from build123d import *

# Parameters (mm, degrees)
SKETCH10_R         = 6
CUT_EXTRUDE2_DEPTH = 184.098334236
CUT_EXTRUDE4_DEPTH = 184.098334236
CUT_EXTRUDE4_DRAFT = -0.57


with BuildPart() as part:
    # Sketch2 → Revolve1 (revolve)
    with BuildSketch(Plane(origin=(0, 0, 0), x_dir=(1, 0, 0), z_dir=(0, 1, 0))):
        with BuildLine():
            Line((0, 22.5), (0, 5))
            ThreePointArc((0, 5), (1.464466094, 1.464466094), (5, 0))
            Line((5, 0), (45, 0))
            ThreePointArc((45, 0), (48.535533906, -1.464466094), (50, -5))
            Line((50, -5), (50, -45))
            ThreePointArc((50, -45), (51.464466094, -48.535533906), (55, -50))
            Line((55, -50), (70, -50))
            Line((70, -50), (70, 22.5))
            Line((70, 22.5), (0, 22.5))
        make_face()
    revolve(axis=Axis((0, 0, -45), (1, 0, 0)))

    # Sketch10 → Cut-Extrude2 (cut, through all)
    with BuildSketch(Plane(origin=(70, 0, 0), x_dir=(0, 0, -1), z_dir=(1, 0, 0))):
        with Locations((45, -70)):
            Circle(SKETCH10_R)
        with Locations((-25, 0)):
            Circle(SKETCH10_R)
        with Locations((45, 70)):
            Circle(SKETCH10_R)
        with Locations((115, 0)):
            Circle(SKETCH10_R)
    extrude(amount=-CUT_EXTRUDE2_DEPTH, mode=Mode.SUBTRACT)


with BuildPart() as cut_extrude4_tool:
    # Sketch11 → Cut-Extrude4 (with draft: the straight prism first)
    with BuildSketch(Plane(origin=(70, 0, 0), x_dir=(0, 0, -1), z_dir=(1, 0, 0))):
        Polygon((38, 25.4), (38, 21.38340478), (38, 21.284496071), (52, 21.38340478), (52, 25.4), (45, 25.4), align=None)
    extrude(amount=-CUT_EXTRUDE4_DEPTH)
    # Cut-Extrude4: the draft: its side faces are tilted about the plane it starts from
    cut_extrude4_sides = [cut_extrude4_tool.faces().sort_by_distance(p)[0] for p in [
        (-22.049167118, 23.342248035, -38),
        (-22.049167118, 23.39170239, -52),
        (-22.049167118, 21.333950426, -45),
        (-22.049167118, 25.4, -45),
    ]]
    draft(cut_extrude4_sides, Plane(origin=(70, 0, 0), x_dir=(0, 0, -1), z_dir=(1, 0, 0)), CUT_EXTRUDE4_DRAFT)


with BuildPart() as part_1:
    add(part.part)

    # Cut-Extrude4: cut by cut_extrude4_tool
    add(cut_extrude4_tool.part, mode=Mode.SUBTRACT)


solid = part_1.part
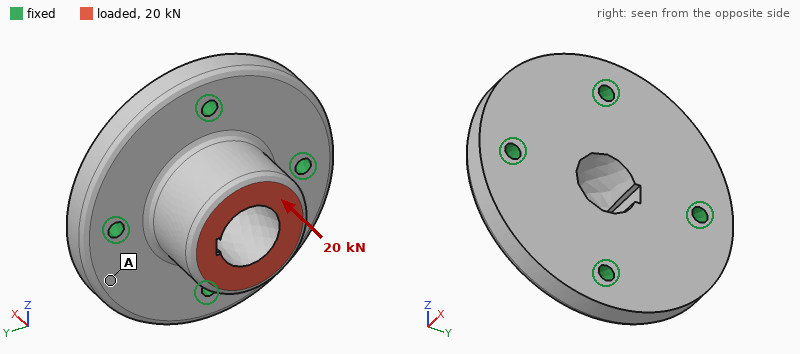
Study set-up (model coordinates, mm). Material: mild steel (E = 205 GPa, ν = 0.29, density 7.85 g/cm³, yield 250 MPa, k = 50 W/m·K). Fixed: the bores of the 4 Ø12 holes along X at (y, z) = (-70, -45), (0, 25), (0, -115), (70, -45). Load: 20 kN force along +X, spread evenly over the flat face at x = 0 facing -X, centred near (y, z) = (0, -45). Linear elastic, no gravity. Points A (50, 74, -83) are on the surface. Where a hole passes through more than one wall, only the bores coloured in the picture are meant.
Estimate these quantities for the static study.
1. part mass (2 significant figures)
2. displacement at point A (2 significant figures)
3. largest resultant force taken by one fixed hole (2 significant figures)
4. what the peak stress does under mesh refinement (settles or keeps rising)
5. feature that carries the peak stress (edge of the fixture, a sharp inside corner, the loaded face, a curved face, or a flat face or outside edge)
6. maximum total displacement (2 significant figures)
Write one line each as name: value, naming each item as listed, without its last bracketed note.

part mass: 6.0 kg
displacement at point A: 0.85 µm
largest resultant force taken by one fixed hole: 5.3 kN
what the peak stress does under mesh refinement: keeps rising
feature that carries the peak stress: edge of the fixture
maximum total displacement: 5.5 µm
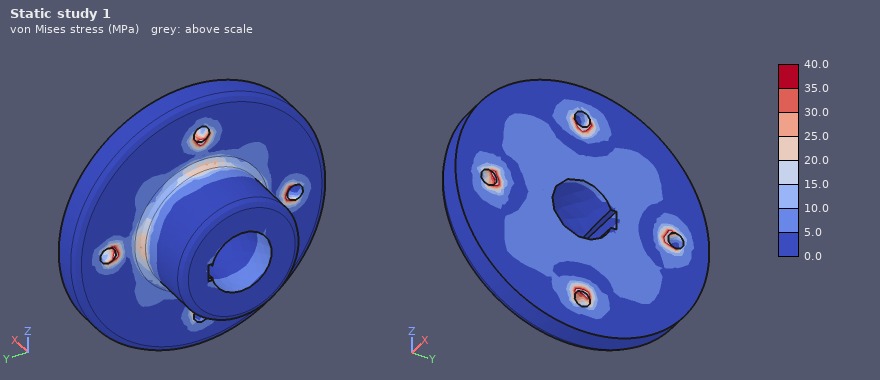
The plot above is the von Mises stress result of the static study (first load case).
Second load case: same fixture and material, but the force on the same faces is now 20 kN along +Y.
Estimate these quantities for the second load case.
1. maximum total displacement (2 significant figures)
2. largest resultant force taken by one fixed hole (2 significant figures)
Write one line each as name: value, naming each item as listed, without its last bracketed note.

maximum total displacement: 17 µm
largest resultant force taken by one fixed hole: 11 kN
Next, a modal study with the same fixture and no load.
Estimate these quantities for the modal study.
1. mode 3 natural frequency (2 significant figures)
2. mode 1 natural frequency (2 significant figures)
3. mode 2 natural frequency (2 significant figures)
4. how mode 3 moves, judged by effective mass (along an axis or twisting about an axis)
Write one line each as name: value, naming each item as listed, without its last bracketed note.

mode 3 natural frequency: 5800 Hz
mode 1 natural frequency: 5500 Hz
mode 2 natural frequency: 5500 Hz
how mode 3 moves, judged by effective mass: along X
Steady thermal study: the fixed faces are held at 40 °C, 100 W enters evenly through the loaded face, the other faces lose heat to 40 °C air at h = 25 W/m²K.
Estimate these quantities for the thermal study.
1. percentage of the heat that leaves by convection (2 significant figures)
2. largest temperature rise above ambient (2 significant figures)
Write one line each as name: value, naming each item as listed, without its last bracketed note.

percentage of the heat that leaves by convection: 20 %
largest temperature rise above ambient: 34 K
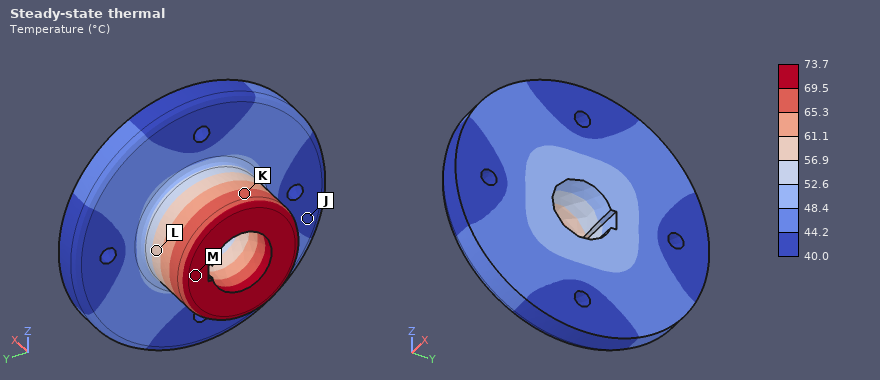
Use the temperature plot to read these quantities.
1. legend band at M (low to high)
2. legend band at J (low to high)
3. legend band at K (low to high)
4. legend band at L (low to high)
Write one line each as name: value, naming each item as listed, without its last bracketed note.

legend band at M: 69.5 to 73.7 °C
legend band at J: 40.0 to 44.2 °C
legend band at K: 65.3 to 69.5 °C
legend band at L: 56.9 to 61.1 °C
